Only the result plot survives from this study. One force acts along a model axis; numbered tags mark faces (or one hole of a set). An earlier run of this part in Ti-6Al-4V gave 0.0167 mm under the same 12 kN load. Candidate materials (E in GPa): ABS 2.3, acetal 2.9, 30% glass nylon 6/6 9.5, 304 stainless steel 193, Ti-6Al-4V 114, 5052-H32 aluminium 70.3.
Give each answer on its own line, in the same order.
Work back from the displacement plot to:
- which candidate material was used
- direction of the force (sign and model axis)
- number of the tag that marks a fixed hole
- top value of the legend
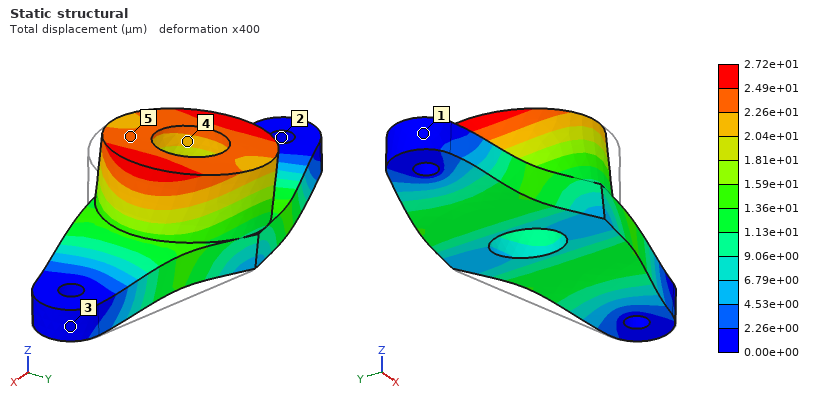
5052-H32 aluminium
-X
2
2.72e+01 µm
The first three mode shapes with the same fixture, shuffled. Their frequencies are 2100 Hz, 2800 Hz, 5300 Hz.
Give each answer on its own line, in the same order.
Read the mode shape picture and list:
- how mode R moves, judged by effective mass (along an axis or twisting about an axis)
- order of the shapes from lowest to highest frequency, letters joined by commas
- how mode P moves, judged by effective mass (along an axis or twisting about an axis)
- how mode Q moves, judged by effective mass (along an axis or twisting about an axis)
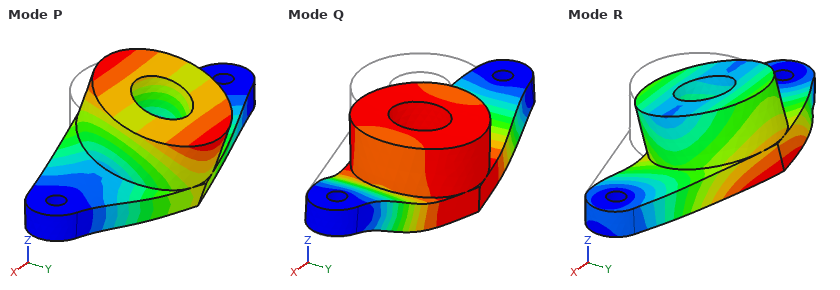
along Y
P, Q, R
along Y
along Z
